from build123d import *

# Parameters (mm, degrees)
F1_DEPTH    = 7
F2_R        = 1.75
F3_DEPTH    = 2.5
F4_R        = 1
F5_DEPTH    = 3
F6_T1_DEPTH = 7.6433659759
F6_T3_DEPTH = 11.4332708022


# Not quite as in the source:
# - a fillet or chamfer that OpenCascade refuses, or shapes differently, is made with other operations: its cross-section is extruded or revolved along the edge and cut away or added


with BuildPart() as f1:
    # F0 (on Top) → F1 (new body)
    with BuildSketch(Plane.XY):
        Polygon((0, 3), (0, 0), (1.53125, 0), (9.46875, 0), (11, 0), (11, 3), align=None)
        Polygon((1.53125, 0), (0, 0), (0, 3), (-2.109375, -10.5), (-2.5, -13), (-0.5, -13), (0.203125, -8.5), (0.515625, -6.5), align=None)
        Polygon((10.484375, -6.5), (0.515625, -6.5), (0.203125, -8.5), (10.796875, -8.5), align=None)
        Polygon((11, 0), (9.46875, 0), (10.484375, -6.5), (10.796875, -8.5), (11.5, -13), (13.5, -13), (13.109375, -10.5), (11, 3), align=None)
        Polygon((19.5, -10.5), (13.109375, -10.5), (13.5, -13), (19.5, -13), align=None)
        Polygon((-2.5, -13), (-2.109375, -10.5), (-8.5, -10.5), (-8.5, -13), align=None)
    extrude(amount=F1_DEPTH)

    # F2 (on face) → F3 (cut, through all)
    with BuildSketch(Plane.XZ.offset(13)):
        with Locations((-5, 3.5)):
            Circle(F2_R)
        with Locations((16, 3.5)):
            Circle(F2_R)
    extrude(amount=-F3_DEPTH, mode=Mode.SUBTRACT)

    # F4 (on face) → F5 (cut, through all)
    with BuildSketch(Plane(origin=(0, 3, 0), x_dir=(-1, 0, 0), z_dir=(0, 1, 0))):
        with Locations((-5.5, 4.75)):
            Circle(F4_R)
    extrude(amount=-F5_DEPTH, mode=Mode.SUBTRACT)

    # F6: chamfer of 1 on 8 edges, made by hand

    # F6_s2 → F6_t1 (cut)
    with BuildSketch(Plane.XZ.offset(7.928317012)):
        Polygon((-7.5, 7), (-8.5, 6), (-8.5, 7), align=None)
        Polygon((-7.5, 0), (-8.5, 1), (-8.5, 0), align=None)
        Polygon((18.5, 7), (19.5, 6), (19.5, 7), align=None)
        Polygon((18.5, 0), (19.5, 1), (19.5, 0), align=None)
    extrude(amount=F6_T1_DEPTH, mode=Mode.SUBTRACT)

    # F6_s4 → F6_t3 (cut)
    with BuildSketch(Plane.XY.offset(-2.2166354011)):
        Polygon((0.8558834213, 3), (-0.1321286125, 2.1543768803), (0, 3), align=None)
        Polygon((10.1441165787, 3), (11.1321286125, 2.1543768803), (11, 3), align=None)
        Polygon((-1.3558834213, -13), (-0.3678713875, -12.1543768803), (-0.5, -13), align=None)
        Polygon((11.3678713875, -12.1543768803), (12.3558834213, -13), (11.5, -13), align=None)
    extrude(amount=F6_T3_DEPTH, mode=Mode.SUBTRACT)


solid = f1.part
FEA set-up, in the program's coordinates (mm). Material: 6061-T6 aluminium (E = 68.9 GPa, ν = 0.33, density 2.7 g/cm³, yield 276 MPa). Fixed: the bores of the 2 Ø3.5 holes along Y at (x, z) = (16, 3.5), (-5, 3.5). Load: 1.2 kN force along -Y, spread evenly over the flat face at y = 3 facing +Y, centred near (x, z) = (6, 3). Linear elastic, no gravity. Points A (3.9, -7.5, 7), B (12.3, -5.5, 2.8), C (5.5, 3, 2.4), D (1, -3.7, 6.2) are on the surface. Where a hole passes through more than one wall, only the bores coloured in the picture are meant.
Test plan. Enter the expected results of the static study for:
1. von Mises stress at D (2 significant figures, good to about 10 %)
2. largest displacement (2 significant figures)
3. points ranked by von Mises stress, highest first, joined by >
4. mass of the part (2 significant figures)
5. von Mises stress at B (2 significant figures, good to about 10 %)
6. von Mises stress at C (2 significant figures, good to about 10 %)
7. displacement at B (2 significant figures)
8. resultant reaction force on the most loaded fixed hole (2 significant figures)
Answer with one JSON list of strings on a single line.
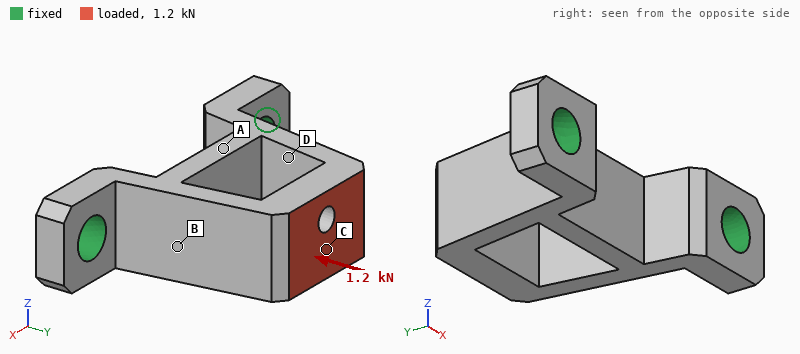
["74 MPa", "27 µm", "C > D > B > A", "2.4 g", "43 MPa", "110 MPa", "11 µm", "630 N"]
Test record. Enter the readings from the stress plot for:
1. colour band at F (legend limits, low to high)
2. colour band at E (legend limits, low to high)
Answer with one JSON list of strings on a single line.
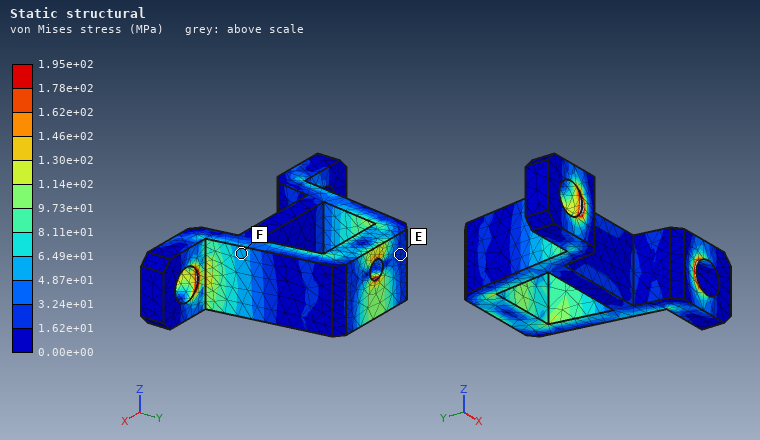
["4.87e+01 to 6.49e+01 MPa", "1.62e+01 to 3.24e+01 MPa"]
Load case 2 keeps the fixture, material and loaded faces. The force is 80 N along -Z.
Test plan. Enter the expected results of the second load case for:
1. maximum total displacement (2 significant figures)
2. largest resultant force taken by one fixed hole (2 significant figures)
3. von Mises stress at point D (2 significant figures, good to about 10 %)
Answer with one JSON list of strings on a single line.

["33 µm", "40 N", "14 MPa"]
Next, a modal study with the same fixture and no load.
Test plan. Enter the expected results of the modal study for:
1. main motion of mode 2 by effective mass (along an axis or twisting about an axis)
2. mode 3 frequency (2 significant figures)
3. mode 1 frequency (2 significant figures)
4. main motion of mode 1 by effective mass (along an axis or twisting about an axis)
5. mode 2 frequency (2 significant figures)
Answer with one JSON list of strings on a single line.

["along X", "22 kHz", "9600 Hz", "along Z", "15 kHz"]
